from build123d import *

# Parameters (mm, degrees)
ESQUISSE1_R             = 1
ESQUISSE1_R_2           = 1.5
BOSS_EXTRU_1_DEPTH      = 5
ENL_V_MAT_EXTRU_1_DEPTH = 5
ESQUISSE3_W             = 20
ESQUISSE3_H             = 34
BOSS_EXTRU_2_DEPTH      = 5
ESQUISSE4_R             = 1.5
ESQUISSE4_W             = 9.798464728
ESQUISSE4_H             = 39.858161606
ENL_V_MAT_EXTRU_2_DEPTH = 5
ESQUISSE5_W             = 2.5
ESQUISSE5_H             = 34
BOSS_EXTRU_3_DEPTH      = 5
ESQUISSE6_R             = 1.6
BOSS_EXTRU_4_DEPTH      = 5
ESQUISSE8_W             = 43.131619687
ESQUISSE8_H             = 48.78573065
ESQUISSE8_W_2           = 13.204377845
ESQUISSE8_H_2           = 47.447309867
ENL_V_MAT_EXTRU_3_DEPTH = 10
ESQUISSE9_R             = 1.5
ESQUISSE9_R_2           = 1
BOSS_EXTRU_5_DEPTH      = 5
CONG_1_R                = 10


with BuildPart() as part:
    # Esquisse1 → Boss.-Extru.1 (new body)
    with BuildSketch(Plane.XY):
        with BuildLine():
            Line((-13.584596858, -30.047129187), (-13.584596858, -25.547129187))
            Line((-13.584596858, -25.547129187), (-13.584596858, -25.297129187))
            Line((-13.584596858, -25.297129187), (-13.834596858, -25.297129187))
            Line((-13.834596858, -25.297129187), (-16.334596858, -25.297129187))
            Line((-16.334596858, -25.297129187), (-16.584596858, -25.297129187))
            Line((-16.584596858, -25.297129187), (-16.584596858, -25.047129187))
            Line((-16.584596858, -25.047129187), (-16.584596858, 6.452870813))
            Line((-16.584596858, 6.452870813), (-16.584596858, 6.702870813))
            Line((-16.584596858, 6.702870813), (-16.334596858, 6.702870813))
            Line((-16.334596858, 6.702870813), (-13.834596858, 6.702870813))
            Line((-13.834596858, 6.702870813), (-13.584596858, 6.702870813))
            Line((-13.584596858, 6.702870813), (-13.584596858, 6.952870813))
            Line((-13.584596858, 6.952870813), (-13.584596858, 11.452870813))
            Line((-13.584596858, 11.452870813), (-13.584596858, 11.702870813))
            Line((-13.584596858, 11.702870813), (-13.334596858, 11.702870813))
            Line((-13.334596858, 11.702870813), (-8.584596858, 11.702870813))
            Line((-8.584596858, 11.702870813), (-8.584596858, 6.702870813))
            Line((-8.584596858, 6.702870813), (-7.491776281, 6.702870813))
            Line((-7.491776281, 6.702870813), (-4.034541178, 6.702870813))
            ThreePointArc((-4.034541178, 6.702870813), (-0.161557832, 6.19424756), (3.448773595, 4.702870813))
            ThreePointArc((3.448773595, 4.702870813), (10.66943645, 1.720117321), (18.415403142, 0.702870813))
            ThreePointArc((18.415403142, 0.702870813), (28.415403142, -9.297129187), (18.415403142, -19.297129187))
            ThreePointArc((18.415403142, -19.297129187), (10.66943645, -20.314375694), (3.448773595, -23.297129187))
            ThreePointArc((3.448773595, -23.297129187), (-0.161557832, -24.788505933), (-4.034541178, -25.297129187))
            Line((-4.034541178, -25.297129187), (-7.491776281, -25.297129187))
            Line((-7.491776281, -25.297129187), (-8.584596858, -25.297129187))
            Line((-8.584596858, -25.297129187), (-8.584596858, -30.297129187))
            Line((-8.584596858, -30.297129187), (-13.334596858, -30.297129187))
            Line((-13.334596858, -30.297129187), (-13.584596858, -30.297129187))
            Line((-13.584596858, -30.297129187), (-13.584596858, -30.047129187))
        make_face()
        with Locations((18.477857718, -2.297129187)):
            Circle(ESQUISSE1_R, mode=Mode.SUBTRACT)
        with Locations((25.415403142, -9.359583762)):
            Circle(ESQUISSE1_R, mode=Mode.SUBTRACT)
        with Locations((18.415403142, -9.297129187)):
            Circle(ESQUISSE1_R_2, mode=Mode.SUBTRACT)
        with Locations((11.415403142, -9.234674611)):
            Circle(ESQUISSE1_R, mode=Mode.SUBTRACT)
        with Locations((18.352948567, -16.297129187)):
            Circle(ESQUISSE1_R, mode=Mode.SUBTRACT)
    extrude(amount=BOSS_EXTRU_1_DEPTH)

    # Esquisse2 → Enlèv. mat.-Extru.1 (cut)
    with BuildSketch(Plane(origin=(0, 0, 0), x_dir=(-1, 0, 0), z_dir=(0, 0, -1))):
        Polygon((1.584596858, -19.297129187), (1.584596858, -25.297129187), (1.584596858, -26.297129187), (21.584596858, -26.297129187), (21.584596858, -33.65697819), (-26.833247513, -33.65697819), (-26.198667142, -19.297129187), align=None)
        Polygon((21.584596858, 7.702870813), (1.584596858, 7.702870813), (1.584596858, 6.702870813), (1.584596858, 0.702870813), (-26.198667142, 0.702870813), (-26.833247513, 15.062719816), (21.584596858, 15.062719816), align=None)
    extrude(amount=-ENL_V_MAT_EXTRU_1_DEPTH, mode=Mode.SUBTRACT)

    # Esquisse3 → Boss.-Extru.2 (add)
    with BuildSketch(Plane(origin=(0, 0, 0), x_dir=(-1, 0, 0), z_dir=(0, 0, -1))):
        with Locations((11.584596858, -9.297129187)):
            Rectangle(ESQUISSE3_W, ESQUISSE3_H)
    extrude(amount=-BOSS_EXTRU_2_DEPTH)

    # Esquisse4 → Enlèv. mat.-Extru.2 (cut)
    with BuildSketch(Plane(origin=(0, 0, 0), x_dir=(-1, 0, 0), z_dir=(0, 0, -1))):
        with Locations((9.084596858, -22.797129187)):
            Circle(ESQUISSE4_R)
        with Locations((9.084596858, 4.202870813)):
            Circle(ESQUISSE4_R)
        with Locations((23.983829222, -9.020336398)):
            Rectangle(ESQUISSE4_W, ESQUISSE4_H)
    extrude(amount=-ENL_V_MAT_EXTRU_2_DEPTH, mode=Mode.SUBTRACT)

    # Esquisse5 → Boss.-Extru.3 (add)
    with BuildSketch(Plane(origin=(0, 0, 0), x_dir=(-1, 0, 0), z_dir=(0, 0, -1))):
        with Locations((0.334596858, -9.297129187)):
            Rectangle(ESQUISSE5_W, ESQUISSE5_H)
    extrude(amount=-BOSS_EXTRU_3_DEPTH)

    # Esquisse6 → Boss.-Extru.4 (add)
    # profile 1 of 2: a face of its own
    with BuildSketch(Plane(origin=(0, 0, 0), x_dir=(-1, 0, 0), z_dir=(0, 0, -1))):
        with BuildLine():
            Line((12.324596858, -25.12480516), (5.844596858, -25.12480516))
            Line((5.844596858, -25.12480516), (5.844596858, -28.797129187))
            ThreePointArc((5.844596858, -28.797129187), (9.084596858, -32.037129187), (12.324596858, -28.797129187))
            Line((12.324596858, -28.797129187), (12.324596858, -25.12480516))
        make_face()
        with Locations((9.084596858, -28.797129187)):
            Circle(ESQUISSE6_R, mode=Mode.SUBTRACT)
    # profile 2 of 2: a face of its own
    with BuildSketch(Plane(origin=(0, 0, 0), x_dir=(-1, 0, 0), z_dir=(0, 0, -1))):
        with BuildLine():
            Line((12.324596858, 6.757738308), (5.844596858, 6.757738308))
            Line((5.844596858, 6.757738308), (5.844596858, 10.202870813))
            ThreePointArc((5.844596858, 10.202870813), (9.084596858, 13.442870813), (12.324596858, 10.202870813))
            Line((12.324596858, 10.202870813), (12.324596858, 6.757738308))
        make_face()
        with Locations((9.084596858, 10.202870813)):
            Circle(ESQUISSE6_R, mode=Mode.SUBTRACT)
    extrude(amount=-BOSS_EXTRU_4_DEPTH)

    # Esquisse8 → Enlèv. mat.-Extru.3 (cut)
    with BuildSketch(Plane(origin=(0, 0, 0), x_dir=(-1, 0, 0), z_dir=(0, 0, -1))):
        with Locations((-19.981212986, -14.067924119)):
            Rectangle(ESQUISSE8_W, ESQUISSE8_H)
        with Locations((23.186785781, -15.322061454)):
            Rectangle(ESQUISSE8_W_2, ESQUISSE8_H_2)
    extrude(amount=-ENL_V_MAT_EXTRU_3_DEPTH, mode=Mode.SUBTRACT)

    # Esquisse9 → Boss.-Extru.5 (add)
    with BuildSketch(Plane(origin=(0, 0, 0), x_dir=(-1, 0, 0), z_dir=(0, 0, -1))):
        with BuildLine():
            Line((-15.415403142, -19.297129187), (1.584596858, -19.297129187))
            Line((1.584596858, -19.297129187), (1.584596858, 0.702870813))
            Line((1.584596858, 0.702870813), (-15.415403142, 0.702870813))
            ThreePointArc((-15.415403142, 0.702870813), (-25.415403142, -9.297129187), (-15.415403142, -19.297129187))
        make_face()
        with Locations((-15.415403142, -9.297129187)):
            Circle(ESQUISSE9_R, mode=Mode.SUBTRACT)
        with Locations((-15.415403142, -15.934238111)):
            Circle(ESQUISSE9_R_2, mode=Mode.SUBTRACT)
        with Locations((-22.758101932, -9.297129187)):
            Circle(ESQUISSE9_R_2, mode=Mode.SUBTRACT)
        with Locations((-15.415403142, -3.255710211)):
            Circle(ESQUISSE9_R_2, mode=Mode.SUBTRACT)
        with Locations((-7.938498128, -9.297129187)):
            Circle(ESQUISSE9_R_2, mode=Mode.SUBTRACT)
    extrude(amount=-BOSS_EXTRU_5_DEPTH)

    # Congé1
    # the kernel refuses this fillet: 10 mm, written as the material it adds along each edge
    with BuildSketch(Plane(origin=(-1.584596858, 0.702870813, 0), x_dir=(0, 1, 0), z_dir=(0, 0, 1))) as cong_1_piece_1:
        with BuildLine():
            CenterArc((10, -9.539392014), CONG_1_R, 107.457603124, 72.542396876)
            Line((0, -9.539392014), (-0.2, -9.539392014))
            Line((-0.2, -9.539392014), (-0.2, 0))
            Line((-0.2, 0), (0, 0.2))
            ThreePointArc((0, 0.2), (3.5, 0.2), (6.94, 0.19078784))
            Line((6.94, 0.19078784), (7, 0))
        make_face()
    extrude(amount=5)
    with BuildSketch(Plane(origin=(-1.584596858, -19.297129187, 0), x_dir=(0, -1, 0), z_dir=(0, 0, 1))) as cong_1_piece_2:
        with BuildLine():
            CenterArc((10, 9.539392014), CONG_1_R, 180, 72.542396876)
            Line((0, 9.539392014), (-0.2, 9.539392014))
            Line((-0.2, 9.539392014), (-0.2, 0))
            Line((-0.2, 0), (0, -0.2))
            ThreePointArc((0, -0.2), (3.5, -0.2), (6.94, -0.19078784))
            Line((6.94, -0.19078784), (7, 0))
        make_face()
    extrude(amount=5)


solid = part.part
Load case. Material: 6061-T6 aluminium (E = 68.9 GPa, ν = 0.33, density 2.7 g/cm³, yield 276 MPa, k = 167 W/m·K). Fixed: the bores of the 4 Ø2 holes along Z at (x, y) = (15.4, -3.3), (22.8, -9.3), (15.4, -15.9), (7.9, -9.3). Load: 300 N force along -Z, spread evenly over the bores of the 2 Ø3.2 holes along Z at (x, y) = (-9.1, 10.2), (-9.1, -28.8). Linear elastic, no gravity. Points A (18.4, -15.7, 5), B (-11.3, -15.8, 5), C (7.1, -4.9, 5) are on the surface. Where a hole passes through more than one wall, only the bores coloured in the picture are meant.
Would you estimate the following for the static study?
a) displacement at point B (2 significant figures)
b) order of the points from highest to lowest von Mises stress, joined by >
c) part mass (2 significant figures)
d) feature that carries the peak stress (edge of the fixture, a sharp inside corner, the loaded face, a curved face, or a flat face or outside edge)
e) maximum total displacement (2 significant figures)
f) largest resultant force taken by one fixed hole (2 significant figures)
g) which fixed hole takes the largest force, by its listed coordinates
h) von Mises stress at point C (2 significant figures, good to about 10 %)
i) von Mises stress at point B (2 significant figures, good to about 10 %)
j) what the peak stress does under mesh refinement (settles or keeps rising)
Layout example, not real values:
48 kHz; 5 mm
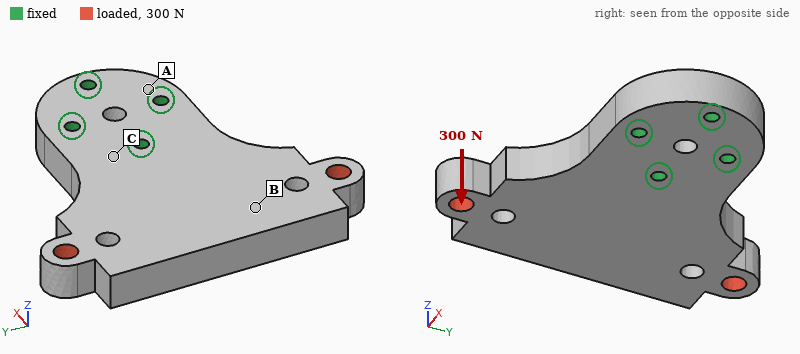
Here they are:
48 µm; C > B > A; 14 g; edge of the fixture; 76 µm; 540 N; (7.9, -9.3); 38 MPa; 19 MPa; keeps rising
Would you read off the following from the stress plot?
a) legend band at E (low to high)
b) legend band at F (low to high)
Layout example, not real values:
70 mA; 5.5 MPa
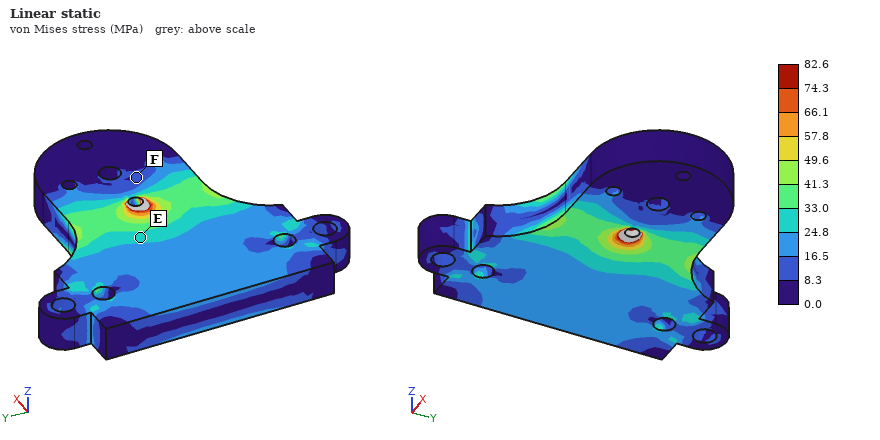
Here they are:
24.8 to 33.0 MPa; 8.3 to 16.5 MPa
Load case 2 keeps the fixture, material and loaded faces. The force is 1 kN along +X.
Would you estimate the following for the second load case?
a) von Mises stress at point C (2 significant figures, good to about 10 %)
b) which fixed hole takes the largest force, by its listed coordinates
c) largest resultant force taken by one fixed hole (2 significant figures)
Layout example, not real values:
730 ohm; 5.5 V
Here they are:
7.6 MPa; (7.9, -9.3); 480 N
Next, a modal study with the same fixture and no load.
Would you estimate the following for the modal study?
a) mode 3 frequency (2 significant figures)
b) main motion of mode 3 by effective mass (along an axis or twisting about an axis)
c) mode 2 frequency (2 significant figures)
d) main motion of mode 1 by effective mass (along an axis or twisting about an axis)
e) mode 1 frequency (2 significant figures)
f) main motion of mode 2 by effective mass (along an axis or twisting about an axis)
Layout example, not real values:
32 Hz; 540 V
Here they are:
10 kHz; along Y; 6100 Hz; along Z; 4600 Hz; twisting about X
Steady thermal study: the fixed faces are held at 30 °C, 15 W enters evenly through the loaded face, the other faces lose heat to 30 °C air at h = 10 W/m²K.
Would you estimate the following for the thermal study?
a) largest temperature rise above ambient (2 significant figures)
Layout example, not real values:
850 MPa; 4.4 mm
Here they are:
26 K
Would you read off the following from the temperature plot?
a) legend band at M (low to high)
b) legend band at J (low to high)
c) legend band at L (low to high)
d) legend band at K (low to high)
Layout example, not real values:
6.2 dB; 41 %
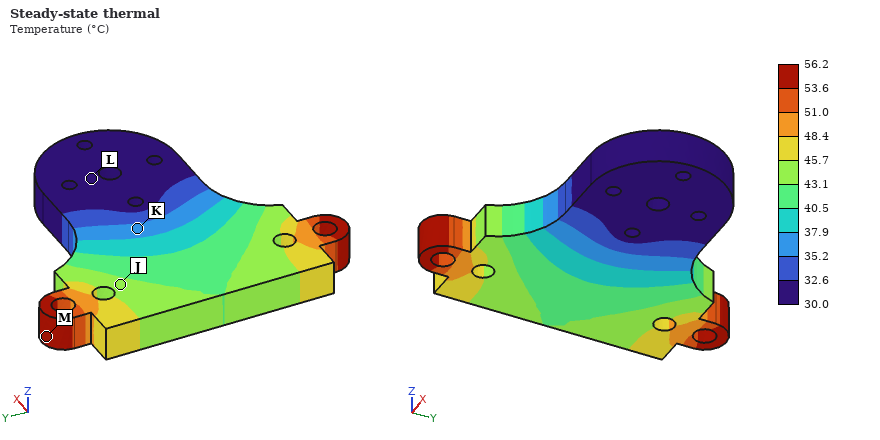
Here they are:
53.6 to 56.2 °C; 43.1 to 45.7 °C; 30.0 to 32.6 °C; 35.2 to 37.9 °C
